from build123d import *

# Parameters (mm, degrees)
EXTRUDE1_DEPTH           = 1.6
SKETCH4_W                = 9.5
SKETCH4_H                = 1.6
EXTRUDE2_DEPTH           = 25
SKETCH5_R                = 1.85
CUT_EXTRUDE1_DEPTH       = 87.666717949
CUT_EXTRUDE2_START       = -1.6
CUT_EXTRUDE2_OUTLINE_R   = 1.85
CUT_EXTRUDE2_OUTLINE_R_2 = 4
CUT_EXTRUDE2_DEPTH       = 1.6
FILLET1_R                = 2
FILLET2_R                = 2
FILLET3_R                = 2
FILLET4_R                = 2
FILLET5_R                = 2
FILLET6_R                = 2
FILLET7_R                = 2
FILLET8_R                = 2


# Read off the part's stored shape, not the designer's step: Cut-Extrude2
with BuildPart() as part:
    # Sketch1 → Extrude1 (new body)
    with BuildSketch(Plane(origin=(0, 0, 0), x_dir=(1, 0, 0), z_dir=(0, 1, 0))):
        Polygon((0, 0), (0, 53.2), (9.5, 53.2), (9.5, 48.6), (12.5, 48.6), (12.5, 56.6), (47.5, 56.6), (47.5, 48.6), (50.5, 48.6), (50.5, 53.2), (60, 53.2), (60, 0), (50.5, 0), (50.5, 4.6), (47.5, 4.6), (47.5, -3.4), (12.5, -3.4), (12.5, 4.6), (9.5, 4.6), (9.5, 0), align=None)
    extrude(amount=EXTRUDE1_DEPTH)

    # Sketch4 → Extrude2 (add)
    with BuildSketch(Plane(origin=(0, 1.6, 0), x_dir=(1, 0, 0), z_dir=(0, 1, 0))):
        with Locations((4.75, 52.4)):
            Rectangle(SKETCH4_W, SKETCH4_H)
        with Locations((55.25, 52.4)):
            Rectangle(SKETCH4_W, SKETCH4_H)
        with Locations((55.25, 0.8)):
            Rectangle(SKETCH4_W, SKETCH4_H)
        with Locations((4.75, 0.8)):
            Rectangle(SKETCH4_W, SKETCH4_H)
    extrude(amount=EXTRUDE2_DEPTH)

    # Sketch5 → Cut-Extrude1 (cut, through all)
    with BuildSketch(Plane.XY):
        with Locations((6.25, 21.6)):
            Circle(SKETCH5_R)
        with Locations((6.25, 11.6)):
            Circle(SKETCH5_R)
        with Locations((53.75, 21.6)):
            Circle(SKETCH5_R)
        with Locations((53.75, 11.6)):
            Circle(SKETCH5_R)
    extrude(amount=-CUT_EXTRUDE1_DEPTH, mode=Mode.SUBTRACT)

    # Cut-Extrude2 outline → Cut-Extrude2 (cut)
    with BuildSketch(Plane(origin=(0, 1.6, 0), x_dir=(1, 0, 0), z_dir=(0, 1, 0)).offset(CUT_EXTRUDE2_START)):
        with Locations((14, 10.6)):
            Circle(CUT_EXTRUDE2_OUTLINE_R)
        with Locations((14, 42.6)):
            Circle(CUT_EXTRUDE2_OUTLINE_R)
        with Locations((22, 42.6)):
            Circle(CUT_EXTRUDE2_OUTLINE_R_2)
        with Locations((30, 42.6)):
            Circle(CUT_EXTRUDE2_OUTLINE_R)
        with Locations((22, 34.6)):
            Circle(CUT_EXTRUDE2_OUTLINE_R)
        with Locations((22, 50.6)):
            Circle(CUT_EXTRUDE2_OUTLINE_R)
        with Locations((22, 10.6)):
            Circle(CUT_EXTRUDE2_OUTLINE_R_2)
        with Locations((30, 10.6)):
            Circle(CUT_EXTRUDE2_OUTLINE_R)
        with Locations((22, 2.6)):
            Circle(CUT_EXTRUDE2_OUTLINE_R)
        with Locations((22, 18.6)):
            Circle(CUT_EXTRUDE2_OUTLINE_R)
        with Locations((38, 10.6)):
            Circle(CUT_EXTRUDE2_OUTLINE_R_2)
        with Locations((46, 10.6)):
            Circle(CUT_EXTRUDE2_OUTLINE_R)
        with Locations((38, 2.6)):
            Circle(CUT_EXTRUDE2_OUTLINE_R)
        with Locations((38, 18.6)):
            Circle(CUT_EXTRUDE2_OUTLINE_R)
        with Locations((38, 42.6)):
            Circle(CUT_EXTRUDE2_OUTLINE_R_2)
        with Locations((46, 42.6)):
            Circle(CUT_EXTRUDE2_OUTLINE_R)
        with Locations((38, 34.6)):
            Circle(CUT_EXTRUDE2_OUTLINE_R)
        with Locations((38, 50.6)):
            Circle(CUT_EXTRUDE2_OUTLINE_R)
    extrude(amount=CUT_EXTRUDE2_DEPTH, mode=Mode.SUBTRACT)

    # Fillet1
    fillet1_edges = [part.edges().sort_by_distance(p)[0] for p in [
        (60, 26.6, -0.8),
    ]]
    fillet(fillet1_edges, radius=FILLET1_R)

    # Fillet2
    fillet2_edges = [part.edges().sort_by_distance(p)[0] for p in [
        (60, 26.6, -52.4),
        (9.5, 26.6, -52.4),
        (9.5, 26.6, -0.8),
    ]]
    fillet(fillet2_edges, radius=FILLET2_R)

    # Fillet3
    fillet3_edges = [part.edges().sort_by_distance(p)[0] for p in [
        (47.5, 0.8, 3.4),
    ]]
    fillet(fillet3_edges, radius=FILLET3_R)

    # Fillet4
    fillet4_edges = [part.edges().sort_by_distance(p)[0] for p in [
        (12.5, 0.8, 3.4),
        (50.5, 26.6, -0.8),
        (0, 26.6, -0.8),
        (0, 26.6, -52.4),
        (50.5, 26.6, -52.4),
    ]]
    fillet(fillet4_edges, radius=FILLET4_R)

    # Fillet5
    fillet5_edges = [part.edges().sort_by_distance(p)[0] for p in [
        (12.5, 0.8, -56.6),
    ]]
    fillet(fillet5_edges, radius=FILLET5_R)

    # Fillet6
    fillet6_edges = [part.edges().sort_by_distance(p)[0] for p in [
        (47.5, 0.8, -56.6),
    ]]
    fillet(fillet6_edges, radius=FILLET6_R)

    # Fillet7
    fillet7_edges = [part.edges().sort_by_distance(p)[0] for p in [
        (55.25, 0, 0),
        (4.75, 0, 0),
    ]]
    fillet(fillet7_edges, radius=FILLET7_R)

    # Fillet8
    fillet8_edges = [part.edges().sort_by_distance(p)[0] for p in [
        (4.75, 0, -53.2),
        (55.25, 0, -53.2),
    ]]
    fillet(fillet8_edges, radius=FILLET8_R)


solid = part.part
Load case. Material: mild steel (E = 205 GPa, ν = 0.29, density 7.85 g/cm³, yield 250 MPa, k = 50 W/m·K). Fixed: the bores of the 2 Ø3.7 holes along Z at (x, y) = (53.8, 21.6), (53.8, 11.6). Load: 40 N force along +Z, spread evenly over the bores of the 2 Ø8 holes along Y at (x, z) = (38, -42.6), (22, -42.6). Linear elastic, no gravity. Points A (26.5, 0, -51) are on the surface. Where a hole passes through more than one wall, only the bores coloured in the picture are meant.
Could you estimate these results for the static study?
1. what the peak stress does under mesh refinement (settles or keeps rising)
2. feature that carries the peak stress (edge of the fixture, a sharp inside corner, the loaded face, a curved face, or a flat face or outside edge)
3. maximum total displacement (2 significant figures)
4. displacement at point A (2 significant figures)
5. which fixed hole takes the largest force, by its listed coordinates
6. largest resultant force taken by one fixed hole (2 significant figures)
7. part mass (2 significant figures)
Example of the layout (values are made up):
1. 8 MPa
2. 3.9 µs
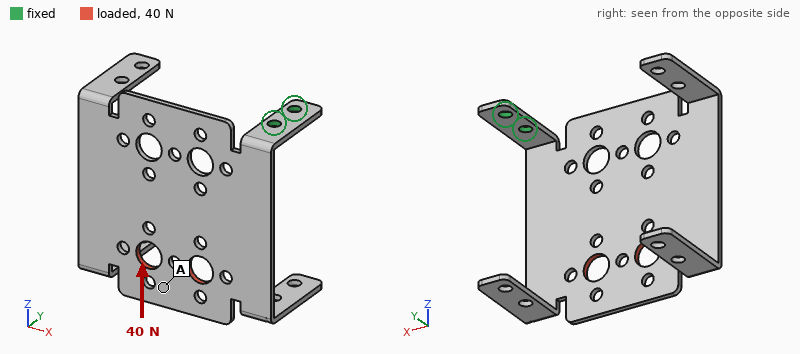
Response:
1. keeps rising
2. edge of the fixture
3. 0.70 mm
4. 0.53 mm
5. (53.8, 11.6)
6. 31 N
7. 48 g
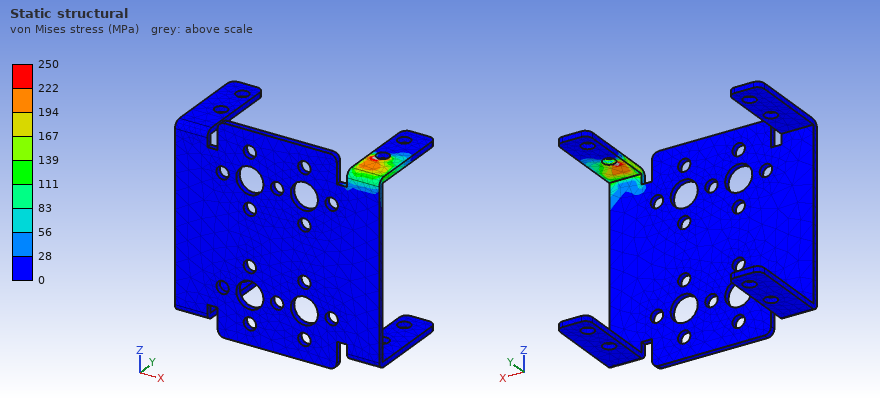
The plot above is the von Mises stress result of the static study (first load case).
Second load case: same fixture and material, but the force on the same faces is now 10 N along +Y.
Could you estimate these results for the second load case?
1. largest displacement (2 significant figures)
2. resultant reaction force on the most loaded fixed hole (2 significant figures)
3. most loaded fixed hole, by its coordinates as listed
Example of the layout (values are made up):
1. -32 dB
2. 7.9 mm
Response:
1. 0.94 mm
2. 22 N
3. (53.8, 11.6)
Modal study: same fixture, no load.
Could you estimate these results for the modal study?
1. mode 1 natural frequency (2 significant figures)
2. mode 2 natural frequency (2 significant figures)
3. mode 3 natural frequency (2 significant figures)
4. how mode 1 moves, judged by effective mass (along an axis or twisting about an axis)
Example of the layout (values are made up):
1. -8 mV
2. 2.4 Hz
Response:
1. 120 Hz
2. 170 Hz
3. 250 Hz
4. along Y
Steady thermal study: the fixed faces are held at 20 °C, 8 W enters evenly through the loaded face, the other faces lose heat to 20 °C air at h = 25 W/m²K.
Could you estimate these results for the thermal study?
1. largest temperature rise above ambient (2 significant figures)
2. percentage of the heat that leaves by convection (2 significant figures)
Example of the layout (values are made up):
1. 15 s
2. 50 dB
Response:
1. 67 K
2. 90 %
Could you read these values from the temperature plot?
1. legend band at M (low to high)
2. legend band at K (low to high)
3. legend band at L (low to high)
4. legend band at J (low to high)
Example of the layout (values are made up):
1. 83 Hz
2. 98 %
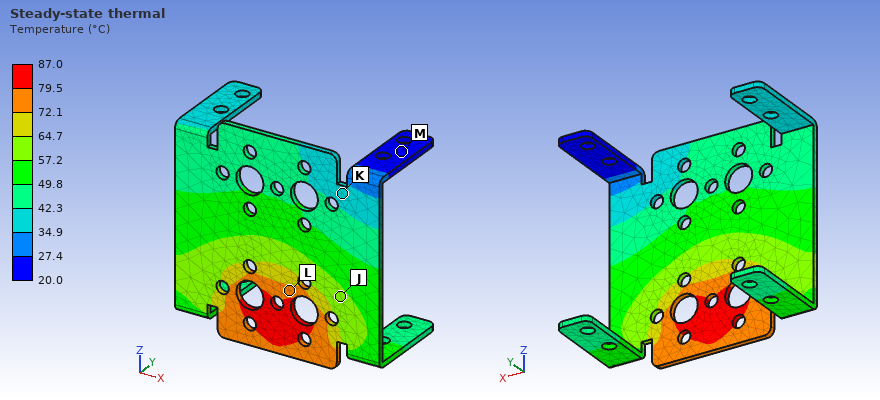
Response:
1. 20.0 to 27.4 °C
2. 34.9 to 42.3 °C
3. 72.1 to 79.5 °C
4. 57.2 to 64.7 °C
